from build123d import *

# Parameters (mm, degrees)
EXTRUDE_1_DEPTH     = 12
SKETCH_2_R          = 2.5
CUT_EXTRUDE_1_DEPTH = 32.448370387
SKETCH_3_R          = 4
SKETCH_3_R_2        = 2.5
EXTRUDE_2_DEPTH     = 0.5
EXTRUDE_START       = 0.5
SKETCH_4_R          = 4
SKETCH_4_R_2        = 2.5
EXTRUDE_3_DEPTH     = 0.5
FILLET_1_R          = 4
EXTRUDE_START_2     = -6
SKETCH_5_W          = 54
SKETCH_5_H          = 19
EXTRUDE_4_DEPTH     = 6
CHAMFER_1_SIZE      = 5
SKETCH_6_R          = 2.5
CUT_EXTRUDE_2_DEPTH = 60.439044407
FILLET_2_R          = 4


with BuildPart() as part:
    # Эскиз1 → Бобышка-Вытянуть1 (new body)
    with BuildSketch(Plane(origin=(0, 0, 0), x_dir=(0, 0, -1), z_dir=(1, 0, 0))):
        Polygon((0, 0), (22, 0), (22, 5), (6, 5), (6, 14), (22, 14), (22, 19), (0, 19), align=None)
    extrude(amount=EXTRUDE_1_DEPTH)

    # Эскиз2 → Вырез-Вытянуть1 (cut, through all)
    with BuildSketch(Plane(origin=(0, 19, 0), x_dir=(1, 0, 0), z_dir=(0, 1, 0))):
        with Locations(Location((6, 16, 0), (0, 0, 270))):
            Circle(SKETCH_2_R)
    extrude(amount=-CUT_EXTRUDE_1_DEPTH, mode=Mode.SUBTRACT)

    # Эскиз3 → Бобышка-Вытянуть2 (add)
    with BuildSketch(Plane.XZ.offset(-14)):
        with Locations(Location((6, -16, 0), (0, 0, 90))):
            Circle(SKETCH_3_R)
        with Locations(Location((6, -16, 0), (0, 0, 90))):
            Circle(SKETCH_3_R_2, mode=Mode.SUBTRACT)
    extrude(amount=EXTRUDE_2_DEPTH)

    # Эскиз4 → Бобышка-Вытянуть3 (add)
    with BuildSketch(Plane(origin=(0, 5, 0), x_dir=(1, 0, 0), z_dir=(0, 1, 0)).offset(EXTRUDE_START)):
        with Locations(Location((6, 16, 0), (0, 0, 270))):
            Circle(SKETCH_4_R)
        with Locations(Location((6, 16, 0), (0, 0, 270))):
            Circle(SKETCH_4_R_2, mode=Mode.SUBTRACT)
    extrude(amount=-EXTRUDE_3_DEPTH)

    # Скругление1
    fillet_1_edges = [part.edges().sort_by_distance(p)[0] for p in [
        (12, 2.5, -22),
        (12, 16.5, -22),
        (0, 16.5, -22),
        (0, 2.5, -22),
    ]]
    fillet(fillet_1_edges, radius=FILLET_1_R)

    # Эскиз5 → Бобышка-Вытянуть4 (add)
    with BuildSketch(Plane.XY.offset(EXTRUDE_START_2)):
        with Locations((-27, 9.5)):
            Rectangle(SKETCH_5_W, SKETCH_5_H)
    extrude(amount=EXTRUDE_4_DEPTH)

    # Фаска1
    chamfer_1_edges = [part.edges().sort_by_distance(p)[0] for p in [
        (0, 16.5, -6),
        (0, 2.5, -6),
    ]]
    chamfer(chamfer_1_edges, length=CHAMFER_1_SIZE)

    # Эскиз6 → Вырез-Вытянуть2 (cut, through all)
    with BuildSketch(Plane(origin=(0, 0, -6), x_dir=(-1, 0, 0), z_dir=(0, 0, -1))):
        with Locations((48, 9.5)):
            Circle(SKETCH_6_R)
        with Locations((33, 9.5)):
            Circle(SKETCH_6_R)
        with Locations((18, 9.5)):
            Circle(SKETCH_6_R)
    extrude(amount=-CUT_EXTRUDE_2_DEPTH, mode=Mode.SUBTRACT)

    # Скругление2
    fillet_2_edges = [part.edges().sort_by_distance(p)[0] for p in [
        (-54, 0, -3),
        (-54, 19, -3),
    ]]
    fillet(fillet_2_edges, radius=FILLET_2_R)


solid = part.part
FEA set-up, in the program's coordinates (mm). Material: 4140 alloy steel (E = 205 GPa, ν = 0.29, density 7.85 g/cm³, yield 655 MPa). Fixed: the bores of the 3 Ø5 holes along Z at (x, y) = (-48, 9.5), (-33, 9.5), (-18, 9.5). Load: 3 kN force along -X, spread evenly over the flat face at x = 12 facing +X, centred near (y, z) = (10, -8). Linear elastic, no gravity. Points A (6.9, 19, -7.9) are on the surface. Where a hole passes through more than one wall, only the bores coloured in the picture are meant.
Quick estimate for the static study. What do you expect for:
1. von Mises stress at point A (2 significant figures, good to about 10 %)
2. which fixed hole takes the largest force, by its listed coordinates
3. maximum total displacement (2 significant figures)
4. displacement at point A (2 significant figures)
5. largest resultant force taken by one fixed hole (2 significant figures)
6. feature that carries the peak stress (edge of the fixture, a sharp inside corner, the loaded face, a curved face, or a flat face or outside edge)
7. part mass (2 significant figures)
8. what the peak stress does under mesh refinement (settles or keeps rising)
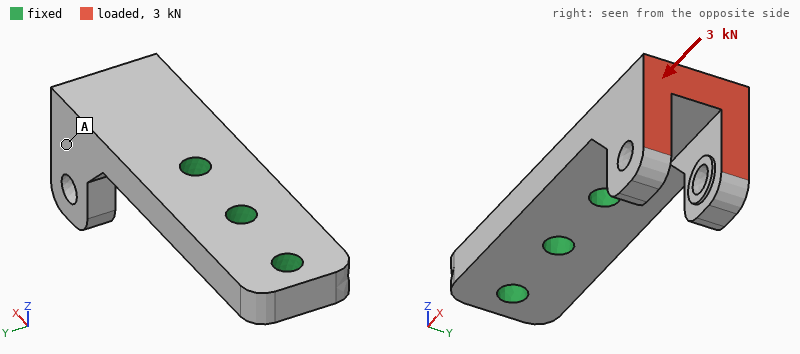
21 MPa
(-18, 9.5)
92 µm
55 µm
2.5 kN
edge of the fixture
70 g
keeps rising
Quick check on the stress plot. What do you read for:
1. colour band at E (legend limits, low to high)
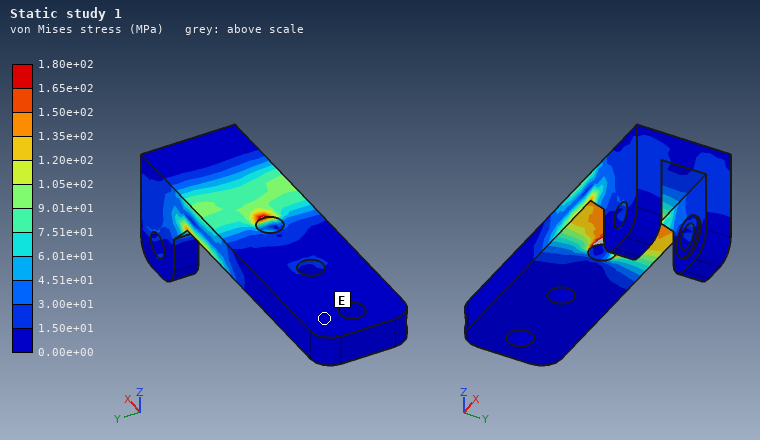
0.00e+00 to 1.50e+01 MPa
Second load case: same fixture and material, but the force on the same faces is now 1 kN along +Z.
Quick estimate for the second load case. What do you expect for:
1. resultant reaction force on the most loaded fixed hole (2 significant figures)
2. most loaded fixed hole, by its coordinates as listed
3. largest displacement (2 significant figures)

1.4 kN
(-18, 9.5)
0.14 mm
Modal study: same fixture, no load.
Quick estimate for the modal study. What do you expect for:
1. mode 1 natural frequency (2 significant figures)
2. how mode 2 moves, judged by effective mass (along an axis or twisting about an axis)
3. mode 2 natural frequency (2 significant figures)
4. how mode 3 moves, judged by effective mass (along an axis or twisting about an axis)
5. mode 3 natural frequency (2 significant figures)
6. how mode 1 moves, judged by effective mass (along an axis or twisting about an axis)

3500 Hz
along Y
5600 Hz
along Y
9400 Hz
along Z
